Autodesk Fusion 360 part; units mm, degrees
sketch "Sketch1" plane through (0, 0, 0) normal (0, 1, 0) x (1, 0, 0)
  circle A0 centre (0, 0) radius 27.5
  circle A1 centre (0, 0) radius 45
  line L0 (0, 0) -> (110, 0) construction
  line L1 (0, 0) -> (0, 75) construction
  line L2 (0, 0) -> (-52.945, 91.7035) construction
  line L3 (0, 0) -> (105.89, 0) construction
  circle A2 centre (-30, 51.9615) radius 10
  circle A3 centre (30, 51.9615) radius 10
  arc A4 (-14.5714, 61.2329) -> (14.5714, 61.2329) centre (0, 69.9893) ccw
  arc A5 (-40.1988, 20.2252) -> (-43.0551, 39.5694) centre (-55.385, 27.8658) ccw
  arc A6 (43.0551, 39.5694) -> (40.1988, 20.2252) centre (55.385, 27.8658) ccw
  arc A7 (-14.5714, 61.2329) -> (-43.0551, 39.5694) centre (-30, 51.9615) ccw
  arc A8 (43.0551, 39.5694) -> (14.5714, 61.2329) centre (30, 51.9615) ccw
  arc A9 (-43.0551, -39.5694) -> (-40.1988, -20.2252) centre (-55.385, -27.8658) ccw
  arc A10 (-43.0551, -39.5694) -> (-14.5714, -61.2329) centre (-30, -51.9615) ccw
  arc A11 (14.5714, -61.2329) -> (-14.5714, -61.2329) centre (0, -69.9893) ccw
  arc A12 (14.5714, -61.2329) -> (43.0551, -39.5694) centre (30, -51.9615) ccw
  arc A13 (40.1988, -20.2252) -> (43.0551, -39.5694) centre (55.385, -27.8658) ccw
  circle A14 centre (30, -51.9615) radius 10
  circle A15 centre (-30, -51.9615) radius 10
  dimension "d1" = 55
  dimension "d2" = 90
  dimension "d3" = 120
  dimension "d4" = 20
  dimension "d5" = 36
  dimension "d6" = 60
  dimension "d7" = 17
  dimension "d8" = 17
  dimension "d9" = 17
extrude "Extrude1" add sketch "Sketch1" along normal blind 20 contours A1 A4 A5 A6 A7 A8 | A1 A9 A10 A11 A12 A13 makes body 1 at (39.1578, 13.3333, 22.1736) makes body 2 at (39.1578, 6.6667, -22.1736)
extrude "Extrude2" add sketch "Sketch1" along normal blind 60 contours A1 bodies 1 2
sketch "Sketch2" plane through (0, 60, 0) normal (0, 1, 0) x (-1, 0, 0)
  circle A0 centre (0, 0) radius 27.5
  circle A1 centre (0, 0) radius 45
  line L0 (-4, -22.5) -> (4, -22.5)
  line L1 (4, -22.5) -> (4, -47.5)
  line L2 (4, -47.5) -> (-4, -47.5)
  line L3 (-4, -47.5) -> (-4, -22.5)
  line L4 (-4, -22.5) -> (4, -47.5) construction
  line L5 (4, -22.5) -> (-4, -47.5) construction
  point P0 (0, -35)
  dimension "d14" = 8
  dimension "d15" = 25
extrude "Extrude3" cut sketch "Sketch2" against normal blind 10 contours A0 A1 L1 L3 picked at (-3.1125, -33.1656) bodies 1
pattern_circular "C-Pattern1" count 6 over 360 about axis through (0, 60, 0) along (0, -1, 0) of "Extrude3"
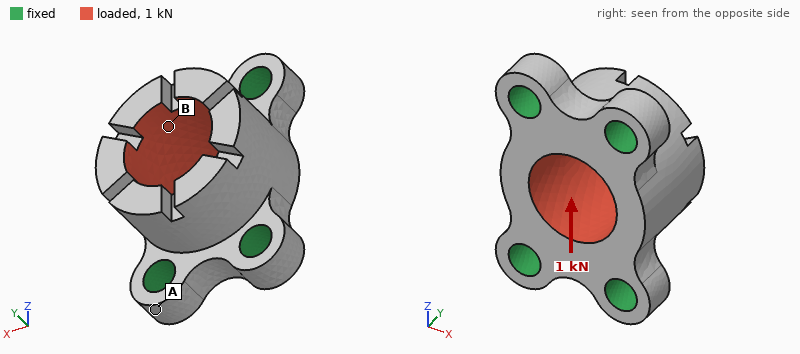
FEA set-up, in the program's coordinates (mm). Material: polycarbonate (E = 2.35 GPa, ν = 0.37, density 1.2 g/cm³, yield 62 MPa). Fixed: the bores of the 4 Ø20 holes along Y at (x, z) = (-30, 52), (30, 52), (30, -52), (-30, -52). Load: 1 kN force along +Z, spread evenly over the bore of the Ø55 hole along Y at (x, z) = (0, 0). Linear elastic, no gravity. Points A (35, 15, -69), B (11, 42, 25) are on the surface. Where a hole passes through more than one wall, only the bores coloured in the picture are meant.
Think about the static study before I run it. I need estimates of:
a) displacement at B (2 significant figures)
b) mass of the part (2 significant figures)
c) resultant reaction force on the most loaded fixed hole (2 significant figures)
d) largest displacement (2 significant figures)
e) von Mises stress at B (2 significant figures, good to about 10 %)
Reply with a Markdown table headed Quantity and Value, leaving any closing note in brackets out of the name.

| Quantity | Value |
|---|---|
| displacement at B | 13 µm |
| mass of the part | 360 g |
| resultant reaction force on the most loaded fixed hole | 280 N |
| largest displacement | 20 µm |
| von Mises stress at B | 0.26 MPa |
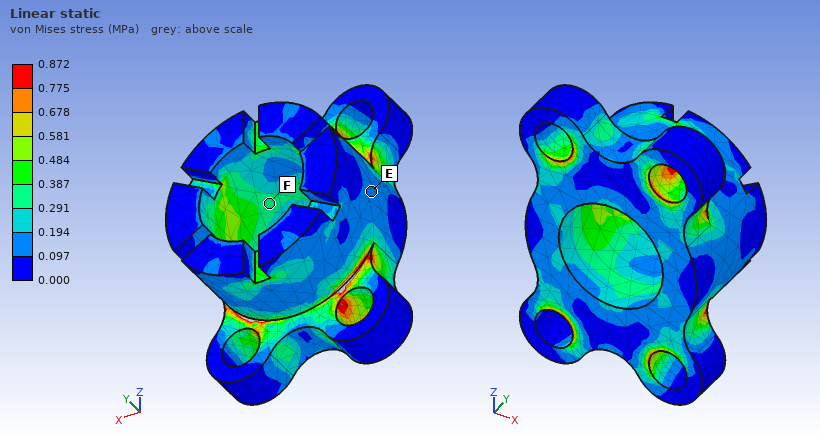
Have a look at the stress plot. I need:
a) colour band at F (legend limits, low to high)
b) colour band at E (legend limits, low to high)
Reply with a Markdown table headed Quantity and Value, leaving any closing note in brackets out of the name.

| Quantity | Value |
|---|---|
| colour band at F | 0.291 to 0.387 MPa |
| colour band at E | 0.097 to 0.194 MPa |
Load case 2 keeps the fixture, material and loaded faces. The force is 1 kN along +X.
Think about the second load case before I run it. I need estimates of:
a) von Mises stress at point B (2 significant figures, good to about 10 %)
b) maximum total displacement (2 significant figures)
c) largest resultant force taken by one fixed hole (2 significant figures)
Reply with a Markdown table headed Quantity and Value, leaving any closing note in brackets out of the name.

| Quantity | Value |
|---|---|
| von Mises stress at point B | 0.53 MPa |
| maximum total displacement | 37 µm |
| largest resultant force taken by one fixed hole | 310 N |
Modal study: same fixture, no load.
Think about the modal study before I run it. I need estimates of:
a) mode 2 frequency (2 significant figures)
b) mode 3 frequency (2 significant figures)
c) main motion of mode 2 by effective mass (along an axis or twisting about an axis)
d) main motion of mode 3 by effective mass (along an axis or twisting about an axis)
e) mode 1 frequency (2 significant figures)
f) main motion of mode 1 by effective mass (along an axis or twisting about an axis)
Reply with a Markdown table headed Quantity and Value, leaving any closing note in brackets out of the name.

| Quantity | Value |
|---|---|
| mode 2 frequency | 2100 Hz |
| mode 3 frequency | 2800 Hz |
| main motion of mode 2 by effective mass | along Y |
| main motion of mode 3 by effective mass | along Z |
| mode 1 frequency | 1900 Hz |
| main motion of mode 1 by effective mass | along X |
